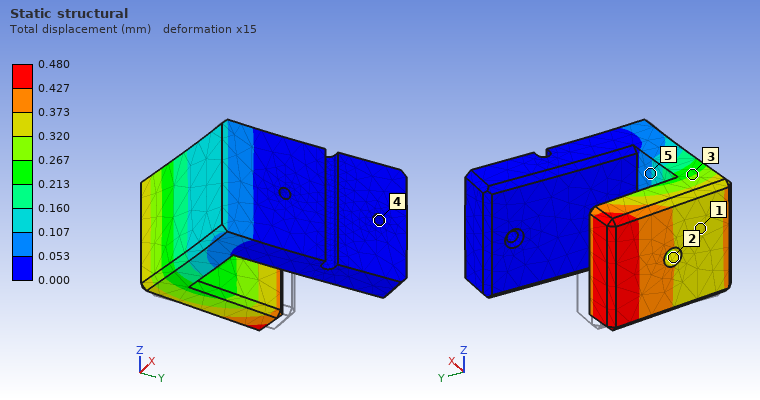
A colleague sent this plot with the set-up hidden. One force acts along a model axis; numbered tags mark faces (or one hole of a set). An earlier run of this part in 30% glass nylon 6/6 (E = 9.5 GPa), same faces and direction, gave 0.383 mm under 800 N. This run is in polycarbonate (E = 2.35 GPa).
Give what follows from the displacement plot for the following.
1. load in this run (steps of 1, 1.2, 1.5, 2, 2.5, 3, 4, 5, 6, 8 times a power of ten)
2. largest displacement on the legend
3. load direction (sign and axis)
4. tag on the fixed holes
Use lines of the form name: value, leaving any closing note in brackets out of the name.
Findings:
load in this run: 250 N
largest displacement on the legend: 0.480 mm
load direction: -Y
tag on the fixed holes: 4
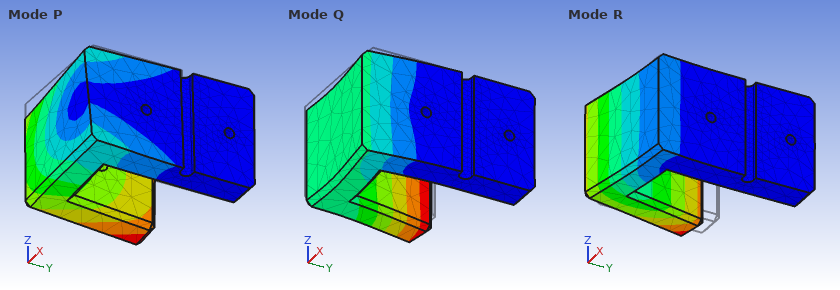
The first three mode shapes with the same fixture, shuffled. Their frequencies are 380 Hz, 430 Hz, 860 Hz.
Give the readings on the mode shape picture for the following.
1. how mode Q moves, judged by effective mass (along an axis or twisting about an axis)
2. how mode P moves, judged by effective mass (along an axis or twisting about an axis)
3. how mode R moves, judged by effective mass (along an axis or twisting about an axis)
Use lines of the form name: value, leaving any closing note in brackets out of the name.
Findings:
how mode Q moves, judged by effective mass: along X
how mode P moves, judged by effective mass: along Z
how mode R moves, judged by effective mass: along Y
